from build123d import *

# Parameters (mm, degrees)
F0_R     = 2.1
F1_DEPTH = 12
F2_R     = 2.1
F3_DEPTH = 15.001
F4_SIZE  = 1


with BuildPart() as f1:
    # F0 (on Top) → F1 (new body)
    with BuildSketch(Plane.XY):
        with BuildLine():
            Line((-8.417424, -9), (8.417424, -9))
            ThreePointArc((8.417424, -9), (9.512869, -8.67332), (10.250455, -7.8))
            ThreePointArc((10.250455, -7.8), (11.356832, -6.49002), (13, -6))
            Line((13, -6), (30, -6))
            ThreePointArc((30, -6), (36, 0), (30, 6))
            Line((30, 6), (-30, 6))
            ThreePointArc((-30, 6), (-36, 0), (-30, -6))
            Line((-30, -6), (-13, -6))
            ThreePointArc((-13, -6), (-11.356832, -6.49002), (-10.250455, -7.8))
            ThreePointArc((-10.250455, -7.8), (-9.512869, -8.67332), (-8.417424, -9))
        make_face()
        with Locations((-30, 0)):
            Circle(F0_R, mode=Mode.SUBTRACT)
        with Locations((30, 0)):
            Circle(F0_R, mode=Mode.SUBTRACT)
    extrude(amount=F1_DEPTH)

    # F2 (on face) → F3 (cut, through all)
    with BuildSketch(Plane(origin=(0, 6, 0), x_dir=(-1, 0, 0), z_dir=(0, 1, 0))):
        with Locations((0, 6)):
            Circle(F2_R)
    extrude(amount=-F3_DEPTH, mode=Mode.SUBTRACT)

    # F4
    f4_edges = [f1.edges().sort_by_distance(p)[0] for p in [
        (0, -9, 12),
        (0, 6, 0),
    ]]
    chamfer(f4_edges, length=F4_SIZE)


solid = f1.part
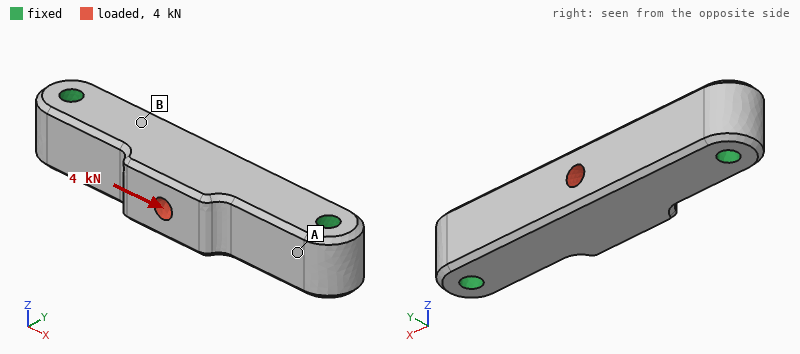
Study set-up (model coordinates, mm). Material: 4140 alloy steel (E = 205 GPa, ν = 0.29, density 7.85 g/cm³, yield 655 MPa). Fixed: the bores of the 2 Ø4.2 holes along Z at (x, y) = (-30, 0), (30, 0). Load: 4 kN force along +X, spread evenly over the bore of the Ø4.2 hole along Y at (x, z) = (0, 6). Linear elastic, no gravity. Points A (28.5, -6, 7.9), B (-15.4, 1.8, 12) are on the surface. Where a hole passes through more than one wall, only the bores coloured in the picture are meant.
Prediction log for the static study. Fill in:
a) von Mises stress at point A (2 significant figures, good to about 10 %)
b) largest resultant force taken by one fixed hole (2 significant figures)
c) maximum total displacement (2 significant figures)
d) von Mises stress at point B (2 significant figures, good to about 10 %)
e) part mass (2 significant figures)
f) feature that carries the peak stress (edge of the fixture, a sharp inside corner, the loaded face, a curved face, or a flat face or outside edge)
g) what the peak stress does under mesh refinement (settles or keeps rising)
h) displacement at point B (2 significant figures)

4.7 MPa
2.0 kN
2.3 µm
13 MPa
79 g
edge of the fixture
keeps rising
1.1 µm
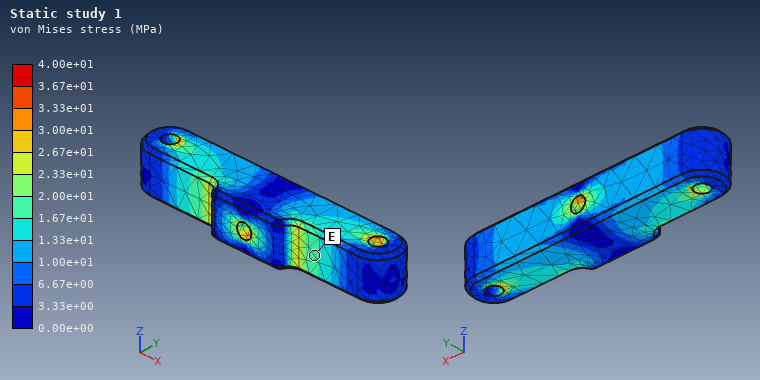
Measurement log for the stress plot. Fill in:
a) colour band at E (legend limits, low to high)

1.67e+01 to 2.00e+01 MPa
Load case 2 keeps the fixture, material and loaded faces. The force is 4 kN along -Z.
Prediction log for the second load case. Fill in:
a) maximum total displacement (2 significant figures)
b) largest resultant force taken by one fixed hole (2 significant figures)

20 µm
2.0 kN
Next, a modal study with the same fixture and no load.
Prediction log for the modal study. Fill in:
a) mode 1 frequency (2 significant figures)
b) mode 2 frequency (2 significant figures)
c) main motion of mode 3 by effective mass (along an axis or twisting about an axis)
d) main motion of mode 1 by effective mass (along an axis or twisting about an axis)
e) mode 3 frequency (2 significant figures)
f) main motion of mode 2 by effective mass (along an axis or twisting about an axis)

13 kHz
14 kHz
twisting about X
along Y
22 kHz
along Z
